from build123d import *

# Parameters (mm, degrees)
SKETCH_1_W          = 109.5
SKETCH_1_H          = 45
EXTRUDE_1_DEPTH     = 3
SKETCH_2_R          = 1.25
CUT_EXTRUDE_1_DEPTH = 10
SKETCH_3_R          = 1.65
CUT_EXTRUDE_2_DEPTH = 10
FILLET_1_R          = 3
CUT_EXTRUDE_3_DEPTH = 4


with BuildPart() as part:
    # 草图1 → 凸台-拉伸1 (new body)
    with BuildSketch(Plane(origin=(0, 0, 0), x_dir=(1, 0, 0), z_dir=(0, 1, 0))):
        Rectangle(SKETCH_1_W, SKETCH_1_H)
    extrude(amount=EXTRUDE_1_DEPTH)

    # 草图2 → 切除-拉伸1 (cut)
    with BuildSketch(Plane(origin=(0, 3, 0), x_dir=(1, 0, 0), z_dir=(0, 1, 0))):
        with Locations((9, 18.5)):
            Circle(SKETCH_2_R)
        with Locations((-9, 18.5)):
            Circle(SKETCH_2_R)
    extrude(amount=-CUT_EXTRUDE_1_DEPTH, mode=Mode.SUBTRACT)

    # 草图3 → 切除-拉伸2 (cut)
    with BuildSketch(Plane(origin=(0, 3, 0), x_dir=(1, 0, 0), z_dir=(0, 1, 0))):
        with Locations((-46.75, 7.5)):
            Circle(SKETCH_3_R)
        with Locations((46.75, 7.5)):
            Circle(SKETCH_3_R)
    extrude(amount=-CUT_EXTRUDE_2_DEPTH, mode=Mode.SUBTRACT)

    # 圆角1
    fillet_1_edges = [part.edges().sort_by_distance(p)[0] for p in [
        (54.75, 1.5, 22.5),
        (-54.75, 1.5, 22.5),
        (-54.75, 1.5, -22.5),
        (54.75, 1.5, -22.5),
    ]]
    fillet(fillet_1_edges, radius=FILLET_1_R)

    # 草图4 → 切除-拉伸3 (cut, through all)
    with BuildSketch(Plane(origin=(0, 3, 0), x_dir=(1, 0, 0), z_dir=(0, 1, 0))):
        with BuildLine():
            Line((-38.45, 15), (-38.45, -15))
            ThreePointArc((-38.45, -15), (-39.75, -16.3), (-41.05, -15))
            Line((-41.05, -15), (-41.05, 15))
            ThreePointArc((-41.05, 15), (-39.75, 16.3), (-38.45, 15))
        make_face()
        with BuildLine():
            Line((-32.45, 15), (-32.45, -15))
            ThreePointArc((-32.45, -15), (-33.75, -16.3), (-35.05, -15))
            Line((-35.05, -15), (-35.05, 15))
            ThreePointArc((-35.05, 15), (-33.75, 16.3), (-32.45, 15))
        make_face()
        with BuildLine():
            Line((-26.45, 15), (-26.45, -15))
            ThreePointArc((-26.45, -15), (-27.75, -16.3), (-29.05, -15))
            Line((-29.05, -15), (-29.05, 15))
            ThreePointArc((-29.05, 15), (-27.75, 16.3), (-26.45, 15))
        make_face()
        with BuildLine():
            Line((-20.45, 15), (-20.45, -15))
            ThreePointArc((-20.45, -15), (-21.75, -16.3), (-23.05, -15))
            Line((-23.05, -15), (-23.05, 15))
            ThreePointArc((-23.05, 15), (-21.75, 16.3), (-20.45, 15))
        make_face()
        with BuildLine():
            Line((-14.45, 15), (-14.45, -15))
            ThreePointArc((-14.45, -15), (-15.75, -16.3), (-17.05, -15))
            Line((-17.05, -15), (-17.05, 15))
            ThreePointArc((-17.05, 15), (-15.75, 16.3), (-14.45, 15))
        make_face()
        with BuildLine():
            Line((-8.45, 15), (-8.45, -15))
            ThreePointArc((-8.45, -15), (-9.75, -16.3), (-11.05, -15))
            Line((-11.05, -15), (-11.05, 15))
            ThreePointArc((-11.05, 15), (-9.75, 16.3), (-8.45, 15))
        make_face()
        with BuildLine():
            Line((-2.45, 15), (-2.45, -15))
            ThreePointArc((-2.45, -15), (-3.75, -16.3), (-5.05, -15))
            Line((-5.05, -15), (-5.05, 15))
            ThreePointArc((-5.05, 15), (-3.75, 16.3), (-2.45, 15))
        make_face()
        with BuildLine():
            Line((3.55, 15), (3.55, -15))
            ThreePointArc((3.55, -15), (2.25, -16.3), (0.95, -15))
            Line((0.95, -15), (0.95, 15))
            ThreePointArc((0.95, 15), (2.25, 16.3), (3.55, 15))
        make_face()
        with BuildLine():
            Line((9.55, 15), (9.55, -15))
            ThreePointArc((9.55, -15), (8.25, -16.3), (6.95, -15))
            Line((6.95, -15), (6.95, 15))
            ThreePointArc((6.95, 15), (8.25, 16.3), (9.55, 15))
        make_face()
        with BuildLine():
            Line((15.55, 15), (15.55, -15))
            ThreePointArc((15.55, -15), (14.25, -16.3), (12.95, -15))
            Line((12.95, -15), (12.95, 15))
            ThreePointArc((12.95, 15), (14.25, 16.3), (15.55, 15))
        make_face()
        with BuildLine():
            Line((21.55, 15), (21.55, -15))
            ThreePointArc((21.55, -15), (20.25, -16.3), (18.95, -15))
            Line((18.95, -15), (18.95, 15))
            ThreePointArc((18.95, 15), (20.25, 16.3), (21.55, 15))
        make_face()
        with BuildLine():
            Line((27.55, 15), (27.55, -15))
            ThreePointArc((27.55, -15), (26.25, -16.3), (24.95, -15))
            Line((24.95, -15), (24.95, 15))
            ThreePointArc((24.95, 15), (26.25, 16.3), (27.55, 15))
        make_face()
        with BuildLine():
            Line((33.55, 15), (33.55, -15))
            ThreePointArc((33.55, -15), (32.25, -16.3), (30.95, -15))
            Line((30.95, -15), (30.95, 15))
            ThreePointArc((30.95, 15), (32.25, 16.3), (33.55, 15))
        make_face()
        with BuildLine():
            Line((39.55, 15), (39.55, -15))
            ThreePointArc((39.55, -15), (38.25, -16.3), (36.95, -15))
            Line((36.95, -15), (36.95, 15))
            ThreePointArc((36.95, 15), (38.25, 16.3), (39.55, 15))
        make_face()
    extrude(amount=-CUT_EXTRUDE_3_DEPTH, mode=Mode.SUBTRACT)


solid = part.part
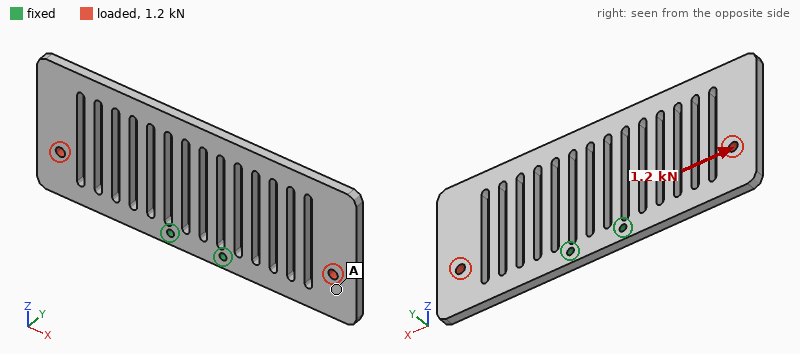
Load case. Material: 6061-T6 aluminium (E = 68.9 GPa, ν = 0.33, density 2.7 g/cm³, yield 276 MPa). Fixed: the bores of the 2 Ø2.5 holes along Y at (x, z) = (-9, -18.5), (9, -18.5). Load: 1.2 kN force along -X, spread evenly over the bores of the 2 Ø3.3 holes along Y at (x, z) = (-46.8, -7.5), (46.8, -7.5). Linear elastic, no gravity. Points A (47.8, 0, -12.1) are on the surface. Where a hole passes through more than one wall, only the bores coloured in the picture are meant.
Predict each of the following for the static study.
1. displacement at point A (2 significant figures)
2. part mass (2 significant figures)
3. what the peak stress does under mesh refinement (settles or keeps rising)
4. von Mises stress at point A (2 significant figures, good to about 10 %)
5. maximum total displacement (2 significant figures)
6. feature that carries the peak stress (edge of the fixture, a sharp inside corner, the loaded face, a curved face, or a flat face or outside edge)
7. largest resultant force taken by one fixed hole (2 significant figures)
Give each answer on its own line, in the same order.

0.21 mm
30 g
keeps rising
23 MPa
0.37 mm
edge of the fixture
810 N
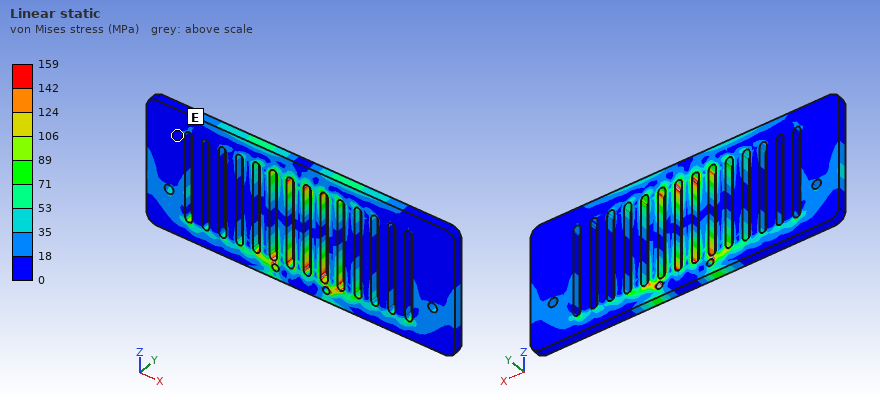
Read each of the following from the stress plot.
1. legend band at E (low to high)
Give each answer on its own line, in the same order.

0 to 18 MPa
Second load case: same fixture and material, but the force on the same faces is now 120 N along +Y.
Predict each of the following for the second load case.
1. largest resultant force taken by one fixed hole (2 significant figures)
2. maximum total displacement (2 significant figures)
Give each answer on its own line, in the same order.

60 N
0.90 mm
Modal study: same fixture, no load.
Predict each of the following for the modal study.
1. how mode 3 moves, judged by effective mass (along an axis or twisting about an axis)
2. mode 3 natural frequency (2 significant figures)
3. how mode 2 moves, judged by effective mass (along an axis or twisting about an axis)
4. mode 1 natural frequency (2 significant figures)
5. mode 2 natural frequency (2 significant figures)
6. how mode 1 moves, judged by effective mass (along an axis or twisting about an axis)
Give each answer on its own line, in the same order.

twisting about X
1100 Hz
along Y
490 Hz
530 Hz
twisting about Z
